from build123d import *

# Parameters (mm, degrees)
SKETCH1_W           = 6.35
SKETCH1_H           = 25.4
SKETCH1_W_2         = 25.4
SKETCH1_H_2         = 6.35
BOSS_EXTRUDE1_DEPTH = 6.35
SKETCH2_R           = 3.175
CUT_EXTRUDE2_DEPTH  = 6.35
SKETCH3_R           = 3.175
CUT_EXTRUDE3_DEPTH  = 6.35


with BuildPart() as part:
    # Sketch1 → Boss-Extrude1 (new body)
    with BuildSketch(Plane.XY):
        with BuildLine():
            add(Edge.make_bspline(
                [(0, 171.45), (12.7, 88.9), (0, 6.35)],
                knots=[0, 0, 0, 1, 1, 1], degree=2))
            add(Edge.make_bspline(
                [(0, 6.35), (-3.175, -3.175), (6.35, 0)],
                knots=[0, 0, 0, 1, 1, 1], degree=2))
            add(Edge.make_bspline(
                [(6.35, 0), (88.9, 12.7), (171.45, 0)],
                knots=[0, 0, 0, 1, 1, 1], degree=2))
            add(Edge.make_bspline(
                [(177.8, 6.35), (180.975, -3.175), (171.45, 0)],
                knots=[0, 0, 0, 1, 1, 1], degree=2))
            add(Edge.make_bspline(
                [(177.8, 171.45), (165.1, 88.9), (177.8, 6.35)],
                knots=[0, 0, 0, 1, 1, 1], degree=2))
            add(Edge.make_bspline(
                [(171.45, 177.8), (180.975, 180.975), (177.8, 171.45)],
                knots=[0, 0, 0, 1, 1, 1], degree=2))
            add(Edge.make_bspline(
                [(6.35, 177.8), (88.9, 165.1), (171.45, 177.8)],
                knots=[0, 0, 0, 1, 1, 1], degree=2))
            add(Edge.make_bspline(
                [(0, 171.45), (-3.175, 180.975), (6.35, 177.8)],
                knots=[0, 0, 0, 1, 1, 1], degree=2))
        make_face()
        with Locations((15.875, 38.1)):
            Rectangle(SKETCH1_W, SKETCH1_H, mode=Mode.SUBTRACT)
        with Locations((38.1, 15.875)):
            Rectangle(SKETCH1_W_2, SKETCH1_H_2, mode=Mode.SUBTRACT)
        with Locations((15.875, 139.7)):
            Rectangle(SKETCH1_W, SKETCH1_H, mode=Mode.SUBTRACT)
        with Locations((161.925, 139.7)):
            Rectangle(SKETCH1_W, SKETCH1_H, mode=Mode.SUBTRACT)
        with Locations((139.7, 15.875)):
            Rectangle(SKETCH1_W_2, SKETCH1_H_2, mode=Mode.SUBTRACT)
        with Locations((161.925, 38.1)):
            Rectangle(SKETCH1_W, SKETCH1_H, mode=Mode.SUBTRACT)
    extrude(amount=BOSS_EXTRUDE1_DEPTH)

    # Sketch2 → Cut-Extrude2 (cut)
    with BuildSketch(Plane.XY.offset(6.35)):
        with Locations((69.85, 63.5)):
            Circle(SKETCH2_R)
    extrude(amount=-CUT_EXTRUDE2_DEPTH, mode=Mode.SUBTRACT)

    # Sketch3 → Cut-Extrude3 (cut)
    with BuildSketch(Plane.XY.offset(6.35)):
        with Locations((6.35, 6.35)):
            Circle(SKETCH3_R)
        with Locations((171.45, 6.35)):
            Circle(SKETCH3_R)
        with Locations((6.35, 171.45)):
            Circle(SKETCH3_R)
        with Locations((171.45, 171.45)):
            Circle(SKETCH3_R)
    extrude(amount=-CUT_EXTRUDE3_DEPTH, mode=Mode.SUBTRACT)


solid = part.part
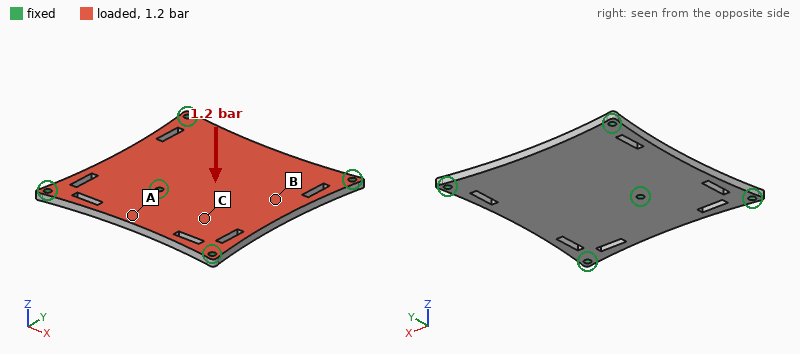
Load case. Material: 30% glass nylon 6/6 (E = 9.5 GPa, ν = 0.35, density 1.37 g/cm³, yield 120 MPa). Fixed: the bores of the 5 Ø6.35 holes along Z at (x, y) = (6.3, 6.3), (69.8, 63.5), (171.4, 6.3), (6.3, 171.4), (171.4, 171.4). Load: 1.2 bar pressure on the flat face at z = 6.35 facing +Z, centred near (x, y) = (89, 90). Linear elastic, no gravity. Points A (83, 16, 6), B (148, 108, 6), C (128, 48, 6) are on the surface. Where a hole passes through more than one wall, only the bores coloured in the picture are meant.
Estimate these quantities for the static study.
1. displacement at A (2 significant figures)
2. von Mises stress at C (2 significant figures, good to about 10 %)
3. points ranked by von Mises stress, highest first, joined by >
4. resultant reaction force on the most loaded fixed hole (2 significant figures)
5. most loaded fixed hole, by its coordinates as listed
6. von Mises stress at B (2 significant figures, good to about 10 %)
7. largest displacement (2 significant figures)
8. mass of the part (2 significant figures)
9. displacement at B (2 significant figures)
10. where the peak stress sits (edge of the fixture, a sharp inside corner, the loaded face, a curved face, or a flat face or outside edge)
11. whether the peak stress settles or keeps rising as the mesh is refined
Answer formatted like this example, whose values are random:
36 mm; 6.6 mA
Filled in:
0.22 mm; 12 MPa; B > C > A; 1.6 kN; (69.8, 63.5); 18 MPa; 1.3 mm; 240 g; 1.1 mm; edge of the fixture; keeps rising
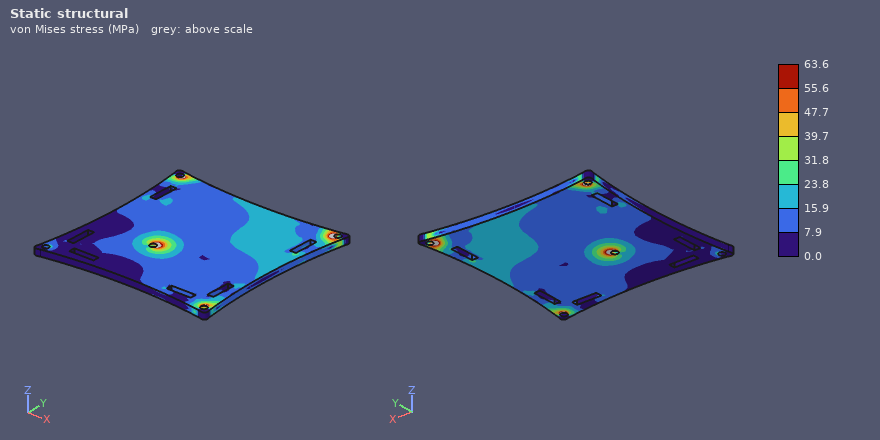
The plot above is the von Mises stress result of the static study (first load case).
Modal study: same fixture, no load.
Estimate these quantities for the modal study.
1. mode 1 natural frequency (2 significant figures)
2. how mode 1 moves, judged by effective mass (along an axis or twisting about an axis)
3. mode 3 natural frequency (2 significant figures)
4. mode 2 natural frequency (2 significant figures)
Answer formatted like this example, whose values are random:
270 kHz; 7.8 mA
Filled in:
600 Hz; along Z; 890 Hz; 730 Hz
